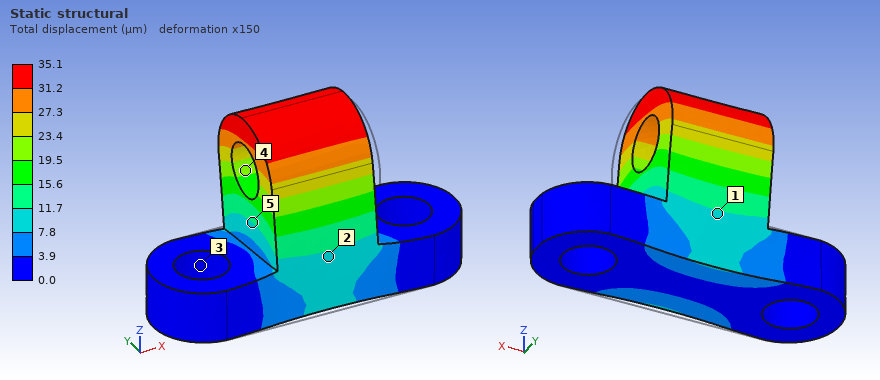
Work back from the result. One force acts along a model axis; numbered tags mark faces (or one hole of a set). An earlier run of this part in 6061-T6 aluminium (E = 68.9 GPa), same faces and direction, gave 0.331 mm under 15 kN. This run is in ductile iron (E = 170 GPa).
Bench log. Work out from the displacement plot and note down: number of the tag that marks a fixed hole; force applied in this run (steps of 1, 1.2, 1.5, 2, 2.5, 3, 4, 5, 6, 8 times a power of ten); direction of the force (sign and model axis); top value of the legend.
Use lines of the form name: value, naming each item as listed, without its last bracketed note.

number of the tag that marks a fixed hole: 3
force applied in this run: 4 kN
direction of the force: +Y
top value of the legend: 35.1 µm
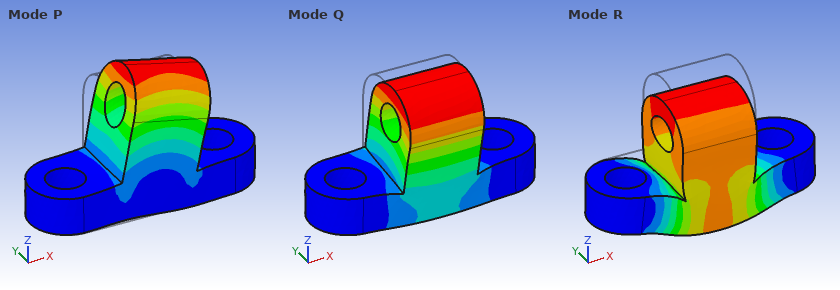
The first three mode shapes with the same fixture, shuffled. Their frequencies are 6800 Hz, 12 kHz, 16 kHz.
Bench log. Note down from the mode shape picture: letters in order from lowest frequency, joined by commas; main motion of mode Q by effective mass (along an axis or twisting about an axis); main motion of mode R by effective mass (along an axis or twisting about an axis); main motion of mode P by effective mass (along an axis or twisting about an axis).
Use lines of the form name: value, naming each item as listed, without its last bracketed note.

letters in order from lowest frequency, joined by commas: Q, P, R
main motion of mode Q by effective mass: along Y
main motion of mode R by effective mass: along Z
main motion of mode P by effective mass: along X
